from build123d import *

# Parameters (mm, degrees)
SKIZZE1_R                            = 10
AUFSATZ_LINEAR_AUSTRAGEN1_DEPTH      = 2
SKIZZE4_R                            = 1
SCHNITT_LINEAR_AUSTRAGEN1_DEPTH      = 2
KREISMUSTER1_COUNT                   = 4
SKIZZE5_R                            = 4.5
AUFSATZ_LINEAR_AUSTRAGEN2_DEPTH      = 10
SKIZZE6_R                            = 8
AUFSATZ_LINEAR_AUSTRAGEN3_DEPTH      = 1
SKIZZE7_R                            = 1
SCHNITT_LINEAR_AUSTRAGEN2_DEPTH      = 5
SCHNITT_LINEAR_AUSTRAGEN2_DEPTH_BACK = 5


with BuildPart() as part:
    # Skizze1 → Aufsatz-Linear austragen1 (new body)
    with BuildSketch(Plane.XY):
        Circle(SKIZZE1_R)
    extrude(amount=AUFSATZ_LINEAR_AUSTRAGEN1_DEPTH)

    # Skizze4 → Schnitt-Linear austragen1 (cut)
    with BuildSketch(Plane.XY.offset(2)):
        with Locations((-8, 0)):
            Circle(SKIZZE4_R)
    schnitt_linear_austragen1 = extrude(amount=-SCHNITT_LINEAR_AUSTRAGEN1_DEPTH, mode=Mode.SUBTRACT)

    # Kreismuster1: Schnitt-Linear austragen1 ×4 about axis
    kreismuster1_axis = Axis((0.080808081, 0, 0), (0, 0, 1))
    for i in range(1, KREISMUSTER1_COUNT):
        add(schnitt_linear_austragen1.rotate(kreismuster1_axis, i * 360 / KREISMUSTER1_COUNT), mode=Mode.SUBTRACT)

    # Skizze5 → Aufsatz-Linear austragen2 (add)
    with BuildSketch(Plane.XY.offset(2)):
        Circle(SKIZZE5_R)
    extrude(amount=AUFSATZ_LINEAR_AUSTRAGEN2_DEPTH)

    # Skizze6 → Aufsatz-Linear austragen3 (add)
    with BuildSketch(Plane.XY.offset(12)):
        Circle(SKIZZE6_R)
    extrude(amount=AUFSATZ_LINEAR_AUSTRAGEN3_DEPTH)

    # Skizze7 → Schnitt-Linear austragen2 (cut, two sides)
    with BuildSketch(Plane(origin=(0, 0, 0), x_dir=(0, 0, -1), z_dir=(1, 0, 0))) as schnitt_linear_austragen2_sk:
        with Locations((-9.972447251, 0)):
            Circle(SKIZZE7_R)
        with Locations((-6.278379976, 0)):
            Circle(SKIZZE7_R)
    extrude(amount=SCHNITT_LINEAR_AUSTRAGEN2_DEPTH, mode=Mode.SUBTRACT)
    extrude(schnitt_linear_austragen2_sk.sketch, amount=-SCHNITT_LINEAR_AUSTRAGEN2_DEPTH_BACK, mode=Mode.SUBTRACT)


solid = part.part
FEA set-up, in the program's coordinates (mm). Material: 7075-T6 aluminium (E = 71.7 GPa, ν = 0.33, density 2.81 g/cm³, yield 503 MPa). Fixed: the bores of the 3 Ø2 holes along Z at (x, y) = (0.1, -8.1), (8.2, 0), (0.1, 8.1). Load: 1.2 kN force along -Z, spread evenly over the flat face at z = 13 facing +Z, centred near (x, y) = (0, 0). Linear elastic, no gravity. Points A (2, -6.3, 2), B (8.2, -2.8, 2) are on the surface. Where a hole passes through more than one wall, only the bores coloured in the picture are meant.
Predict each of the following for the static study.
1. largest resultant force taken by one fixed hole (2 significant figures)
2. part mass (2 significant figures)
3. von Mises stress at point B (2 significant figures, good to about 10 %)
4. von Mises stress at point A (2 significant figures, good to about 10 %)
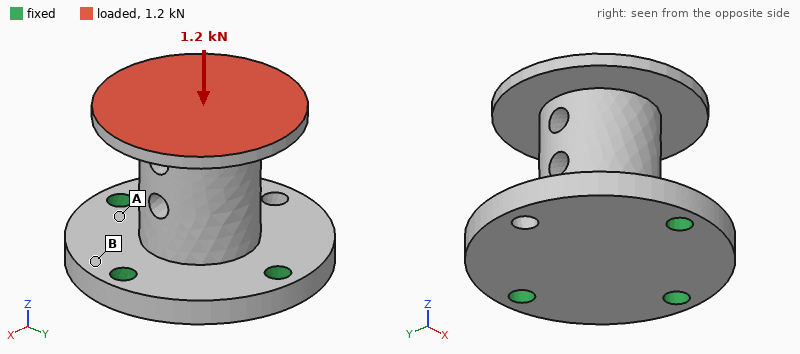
540 N
3.9 g
27 MPa
52 MPa
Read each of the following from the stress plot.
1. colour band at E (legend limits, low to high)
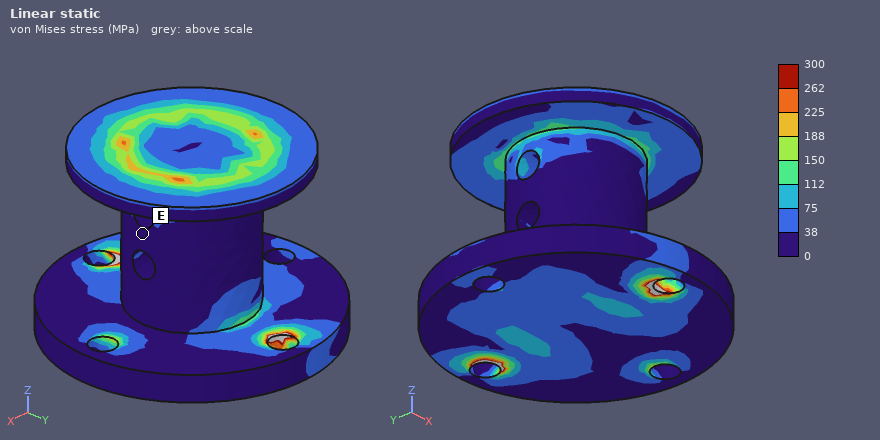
0 to 38 MPa
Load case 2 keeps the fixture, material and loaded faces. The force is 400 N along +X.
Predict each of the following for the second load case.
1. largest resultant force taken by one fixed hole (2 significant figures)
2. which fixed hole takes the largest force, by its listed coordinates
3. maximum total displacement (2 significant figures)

550 N
(8.2, 0)
94 µm
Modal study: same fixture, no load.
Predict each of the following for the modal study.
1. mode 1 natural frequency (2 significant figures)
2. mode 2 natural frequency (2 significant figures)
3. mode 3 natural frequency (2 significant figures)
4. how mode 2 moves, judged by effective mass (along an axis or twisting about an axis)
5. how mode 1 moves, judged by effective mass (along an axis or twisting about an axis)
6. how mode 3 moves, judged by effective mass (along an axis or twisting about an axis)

10 kHz
16 kHz
26 kHz
along Y
along X
along Z
